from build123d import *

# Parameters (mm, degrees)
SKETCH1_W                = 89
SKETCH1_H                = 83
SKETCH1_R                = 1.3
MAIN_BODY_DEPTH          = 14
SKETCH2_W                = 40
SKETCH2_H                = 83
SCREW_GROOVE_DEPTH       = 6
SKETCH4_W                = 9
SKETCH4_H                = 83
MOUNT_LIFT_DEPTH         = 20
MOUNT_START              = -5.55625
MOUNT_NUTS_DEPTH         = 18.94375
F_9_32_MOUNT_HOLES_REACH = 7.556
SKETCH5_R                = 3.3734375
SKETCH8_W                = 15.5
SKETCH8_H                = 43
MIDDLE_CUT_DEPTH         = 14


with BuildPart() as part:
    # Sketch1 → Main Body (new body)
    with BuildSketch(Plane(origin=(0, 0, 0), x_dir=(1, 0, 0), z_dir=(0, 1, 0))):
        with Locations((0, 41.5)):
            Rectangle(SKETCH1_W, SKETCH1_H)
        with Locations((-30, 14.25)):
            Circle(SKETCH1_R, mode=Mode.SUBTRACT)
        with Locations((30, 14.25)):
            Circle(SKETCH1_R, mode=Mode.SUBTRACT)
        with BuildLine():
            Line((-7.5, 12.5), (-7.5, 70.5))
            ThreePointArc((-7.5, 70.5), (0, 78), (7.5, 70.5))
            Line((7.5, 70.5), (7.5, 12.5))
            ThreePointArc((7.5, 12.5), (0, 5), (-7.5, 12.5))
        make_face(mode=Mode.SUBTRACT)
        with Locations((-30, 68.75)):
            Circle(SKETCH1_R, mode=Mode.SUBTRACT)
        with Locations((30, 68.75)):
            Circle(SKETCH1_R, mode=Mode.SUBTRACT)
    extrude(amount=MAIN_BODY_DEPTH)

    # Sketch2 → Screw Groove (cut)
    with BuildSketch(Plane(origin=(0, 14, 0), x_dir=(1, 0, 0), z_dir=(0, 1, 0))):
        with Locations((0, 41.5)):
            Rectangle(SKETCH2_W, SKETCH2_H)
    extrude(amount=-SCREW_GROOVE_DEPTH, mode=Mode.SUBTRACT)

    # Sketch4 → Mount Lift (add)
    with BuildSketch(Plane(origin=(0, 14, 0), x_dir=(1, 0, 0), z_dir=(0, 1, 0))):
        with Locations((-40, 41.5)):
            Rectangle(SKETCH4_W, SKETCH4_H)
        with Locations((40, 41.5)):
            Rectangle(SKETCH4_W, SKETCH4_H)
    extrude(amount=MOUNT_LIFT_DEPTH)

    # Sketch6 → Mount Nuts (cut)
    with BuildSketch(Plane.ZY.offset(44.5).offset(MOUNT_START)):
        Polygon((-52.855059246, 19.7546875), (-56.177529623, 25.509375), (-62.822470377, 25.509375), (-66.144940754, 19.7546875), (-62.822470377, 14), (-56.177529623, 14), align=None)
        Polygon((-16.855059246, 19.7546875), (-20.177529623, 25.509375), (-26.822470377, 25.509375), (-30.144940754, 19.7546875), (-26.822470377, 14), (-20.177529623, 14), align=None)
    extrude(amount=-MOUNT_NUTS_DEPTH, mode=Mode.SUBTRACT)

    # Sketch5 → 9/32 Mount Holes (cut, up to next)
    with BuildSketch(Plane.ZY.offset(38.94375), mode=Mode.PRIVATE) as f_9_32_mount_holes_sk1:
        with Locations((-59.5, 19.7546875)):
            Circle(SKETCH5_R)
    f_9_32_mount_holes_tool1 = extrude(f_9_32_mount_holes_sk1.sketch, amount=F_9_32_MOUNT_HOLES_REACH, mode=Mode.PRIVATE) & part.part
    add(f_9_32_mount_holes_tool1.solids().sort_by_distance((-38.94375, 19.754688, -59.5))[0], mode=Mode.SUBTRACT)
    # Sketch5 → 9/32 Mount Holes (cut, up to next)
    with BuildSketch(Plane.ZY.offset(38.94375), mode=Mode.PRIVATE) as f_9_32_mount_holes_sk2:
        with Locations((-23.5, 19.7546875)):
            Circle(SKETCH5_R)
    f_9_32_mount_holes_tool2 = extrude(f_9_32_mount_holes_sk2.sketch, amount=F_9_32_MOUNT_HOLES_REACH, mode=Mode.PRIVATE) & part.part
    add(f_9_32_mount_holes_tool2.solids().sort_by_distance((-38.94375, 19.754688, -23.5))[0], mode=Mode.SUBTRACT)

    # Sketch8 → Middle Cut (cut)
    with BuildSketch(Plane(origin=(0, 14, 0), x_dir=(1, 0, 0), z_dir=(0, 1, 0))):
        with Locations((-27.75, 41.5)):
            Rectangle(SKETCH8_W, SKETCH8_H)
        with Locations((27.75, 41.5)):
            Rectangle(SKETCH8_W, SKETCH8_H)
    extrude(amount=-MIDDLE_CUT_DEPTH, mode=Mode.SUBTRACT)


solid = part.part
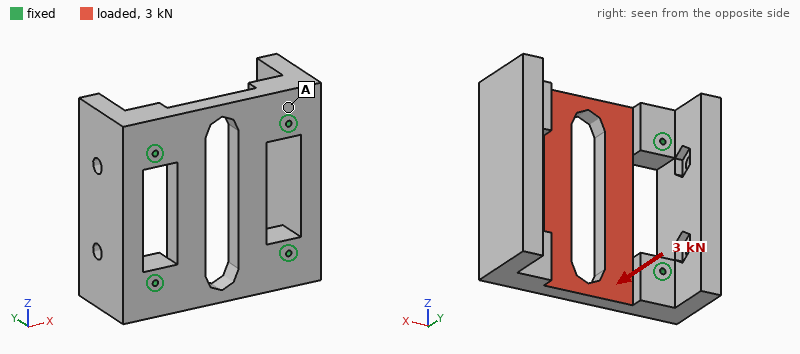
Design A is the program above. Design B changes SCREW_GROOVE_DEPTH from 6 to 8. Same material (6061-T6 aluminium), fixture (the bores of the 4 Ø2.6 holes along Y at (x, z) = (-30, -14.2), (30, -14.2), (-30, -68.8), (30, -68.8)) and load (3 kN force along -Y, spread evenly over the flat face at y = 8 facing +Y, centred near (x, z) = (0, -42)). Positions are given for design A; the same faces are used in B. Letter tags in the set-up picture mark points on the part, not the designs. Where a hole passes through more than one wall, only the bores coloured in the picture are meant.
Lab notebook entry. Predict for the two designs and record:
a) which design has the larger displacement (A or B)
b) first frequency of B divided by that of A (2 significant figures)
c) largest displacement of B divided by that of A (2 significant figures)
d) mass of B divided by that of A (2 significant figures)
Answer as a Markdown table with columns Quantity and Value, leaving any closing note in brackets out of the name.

| Quantity | Value |
|---|---|
| which design has the larger displacement | B |
| first frequency of B divided by that of A | 1.00 |
| largest displacement of B divided by that of A | 1.8 |
| mass of B divided by that of A | 0.95 |
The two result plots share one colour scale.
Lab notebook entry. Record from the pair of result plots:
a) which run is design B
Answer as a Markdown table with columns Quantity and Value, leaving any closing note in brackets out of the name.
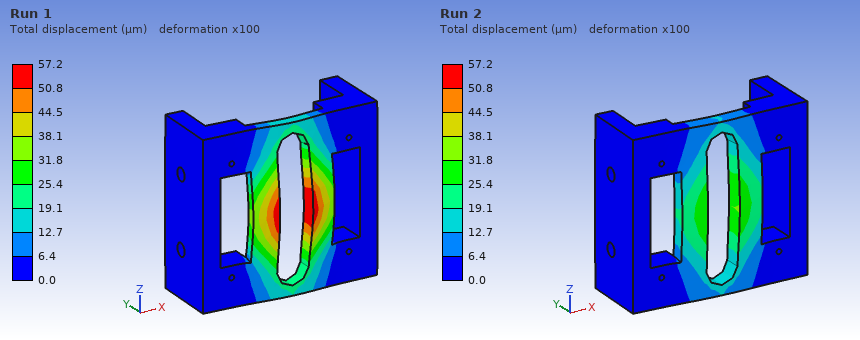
| Quantity | Value |
|---|---|
| which run is design B | Run 1 |
